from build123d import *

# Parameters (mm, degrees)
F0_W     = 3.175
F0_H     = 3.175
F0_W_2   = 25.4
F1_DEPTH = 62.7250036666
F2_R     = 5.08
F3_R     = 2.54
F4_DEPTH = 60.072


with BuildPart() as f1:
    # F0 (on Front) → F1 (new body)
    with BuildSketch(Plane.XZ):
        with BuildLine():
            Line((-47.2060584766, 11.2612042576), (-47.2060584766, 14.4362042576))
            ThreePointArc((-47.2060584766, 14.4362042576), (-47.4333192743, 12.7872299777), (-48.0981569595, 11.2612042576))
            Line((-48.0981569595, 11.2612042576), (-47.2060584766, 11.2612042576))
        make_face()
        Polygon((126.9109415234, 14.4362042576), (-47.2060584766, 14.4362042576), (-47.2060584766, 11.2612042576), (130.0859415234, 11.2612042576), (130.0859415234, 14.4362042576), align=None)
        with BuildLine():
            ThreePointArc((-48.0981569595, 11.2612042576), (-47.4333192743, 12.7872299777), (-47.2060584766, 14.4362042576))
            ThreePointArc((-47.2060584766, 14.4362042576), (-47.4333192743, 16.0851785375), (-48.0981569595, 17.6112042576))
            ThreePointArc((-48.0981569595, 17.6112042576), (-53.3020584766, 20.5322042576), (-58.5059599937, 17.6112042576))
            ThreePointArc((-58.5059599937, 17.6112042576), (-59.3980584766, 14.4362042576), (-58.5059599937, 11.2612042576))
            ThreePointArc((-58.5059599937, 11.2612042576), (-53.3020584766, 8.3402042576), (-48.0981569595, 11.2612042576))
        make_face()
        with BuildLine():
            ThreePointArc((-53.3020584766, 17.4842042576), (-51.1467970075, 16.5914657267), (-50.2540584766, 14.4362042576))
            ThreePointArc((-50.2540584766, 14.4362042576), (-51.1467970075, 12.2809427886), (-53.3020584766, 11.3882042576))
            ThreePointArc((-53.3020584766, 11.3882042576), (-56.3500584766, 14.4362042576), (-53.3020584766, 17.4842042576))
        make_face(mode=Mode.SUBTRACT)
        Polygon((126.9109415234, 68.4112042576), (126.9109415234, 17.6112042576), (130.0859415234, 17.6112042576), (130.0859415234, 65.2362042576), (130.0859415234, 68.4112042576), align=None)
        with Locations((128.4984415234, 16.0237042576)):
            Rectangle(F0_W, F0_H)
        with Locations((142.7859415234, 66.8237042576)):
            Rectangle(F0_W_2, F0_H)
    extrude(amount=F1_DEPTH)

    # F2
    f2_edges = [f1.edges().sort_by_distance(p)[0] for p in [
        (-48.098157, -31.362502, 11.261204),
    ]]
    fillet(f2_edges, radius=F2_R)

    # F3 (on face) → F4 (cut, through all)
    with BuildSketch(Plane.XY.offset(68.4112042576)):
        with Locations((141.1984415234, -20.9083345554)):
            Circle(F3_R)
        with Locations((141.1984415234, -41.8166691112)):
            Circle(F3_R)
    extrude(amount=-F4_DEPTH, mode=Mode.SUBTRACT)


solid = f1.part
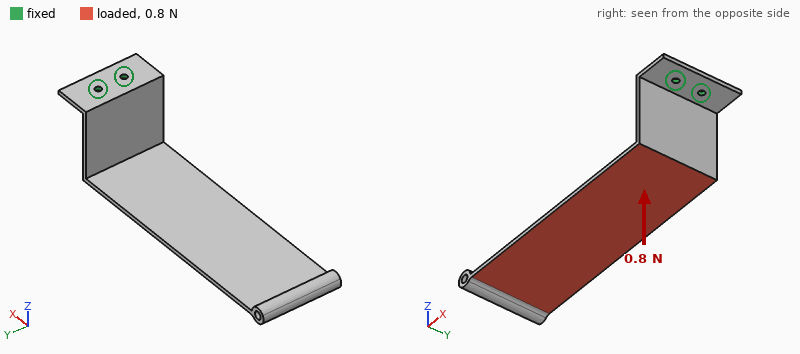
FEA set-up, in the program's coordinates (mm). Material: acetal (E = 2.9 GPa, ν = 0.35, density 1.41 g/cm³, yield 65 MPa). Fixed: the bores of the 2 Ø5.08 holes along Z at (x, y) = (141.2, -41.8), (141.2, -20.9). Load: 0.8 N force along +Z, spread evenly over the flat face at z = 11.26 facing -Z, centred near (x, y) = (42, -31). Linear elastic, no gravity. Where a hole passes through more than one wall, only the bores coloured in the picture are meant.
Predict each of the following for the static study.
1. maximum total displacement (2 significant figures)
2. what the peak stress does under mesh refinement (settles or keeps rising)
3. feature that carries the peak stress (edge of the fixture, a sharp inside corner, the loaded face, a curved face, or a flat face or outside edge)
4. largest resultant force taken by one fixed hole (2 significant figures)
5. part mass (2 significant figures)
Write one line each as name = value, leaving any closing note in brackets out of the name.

maximum total displacement = 2.8 mm
what the peak stress does under mesh refinement = keeps rising
feature that carries the peak stress = edge of the fixture
largest resultant force taken by one fixed hole = 0.44 N
part mass = 80 g
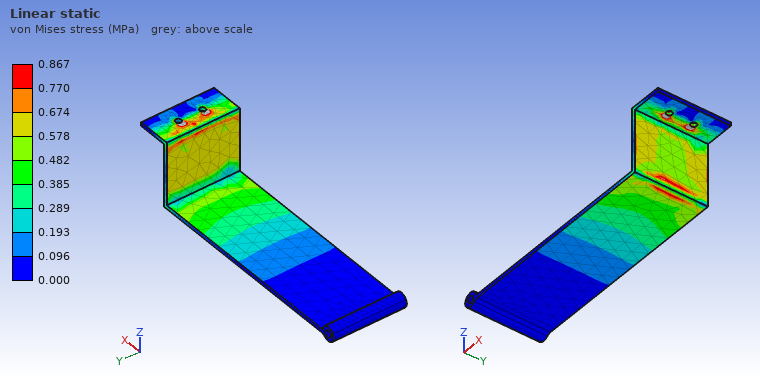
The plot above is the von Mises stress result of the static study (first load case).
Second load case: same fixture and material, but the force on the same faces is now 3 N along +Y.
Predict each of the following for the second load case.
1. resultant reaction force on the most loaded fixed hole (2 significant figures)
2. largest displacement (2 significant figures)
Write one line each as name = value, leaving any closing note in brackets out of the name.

resultant reaction force on the most loaded fixed hole = 13 N
largest displacement = 2.4 mm
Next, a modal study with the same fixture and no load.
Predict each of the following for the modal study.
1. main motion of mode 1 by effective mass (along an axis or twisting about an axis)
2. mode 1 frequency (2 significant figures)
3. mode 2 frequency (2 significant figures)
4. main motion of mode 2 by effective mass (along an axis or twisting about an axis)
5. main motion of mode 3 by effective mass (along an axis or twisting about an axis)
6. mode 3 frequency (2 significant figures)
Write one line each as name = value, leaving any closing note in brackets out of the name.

main motion of mode 1 by effective mass = along Z
mode 1 frequency = 12 Hz
mode 2 frequency = 25 Hz
main motion of mode 2 by effective mass = along Y
main motion of mode 3 by effective mass = along X
mode 3 frequency = 62 Hz
